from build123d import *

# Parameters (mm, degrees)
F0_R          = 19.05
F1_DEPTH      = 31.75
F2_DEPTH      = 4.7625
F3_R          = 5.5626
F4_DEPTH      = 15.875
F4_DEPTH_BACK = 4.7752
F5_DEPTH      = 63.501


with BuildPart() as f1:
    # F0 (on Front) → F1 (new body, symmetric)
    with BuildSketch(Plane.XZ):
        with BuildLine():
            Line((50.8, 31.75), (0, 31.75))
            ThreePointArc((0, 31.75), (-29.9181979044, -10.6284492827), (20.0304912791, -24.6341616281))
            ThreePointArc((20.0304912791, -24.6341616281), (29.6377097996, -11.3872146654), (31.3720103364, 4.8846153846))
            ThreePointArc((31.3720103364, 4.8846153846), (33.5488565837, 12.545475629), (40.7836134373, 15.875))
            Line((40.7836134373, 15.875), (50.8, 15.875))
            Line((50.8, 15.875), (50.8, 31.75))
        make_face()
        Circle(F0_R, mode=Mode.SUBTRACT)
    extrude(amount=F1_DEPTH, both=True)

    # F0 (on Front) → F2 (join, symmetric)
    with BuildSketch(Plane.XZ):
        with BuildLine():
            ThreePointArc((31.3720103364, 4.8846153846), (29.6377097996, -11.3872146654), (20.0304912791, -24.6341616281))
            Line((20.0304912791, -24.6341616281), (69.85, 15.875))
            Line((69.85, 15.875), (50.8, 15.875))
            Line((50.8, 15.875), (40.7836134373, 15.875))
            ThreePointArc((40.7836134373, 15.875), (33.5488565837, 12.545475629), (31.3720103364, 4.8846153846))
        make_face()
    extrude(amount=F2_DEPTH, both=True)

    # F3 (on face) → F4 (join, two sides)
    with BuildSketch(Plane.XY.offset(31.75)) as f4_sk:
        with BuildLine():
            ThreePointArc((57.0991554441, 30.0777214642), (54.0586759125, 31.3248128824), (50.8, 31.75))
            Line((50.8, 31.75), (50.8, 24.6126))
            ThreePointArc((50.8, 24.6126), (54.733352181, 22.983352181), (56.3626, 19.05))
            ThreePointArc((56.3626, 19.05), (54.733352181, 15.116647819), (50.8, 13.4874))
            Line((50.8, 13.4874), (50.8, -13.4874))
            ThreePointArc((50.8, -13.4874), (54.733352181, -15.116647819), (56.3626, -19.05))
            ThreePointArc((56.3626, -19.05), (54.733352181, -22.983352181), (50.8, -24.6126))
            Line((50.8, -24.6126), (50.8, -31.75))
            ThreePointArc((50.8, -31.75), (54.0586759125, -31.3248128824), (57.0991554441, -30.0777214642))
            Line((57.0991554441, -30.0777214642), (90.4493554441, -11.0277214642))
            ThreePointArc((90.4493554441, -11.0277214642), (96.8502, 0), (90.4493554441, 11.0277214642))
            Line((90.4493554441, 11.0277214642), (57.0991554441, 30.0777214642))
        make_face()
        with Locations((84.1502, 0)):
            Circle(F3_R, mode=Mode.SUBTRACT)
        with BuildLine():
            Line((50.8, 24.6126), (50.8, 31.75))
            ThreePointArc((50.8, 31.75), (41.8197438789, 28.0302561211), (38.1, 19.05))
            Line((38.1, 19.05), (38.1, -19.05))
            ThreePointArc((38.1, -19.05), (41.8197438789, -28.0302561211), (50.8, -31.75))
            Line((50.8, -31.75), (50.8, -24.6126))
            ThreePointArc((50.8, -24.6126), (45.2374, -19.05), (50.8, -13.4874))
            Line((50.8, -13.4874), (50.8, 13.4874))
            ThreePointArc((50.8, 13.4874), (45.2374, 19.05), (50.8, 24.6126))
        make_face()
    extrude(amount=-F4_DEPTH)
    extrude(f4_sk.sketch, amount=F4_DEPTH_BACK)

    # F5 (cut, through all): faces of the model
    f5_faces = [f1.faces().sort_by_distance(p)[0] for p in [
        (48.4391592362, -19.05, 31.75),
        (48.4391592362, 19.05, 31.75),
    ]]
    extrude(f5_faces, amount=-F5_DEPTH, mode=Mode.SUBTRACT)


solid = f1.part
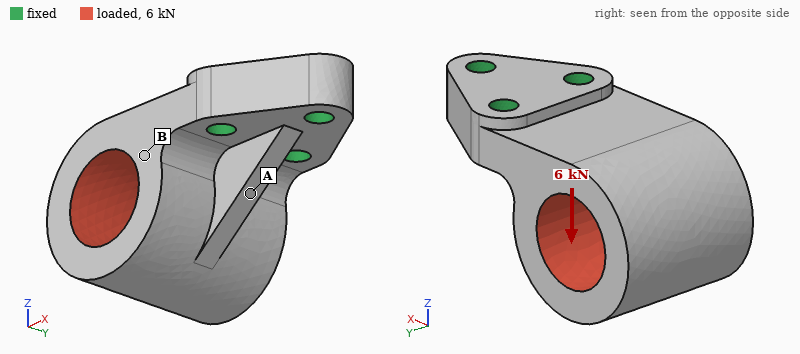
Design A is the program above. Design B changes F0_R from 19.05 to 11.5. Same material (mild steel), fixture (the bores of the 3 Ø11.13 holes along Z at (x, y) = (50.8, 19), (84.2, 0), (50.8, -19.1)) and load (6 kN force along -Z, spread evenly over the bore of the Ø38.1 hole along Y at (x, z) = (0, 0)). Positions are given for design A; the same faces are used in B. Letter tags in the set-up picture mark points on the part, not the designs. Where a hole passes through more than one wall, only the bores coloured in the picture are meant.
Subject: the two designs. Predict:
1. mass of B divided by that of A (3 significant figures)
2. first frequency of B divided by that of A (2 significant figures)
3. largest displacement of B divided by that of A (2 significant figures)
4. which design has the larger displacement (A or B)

1.23
0.93
0.89
A
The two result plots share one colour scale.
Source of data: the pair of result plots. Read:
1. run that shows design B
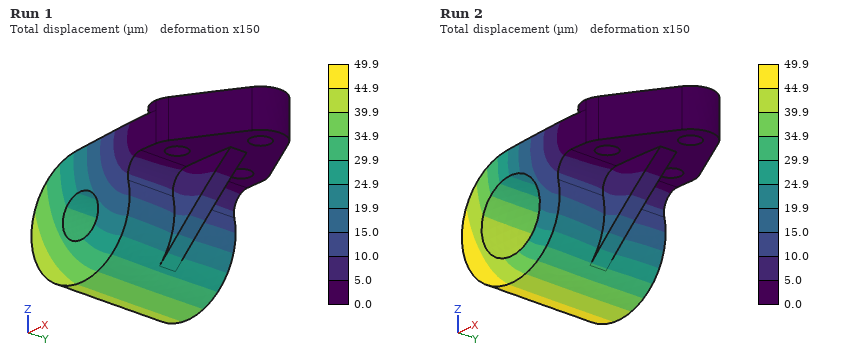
Run 1
